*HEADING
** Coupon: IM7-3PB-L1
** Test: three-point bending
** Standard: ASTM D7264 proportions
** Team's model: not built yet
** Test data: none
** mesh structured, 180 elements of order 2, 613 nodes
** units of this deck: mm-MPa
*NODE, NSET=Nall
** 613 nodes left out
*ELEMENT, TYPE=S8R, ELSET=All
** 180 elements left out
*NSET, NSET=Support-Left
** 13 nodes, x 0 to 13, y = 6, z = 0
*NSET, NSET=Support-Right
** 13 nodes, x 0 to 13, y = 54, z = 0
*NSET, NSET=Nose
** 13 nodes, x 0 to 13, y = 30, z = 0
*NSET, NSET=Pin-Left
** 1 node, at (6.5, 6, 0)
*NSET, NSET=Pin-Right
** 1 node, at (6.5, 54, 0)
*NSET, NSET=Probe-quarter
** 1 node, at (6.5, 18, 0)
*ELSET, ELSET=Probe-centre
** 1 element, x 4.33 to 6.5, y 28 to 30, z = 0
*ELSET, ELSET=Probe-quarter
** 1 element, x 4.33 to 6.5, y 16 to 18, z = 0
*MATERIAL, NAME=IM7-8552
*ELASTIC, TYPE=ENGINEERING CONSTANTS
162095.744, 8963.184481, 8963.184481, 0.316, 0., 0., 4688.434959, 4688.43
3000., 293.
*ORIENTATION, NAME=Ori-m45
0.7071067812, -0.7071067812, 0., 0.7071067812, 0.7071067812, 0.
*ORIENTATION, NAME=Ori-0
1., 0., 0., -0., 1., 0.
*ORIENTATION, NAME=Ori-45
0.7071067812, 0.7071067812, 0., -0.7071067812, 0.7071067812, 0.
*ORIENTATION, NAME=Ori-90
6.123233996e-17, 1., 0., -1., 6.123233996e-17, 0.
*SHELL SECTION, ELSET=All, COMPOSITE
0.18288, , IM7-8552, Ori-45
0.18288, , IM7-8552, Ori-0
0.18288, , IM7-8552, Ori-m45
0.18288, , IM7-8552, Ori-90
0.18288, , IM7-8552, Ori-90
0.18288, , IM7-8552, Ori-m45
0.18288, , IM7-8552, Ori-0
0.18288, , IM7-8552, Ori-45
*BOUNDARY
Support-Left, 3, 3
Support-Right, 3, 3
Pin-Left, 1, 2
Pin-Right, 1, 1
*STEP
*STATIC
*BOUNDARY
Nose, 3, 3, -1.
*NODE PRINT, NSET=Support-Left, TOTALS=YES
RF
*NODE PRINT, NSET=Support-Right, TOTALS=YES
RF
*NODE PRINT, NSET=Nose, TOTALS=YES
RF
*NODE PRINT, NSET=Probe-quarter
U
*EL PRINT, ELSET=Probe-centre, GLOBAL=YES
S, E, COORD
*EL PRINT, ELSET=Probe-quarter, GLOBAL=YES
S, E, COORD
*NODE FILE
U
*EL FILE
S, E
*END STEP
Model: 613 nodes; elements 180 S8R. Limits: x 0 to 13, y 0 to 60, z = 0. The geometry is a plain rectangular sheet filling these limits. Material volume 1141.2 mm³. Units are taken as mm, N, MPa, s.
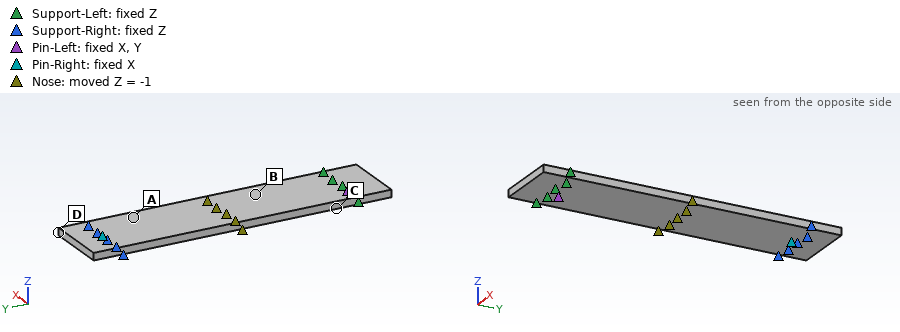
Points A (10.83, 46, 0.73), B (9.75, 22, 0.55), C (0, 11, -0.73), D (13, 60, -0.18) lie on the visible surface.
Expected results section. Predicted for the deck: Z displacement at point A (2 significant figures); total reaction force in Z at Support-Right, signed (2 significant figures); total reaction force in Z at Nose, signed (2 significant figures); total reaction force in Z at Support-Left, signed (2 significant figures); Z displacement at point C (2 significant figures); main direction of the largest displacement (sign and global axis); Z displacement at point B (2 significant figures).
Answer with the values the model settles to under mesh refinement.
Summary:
-0.49 mm
21 N
-43 N
21 N
-0.32 mm
-Z
-0.84 mm
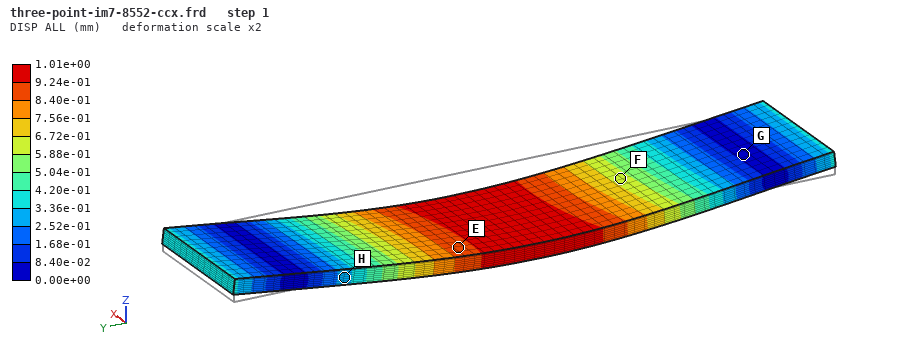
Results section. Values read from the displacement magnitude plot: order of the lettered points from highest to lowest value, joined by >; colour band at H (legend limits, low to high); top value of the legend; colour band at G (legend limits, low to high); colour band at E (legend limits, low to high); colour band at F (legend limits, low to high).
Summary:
E > F > H > G
2.52e-01 to 3.36e-01 mm
1.01e+00 mm
0.00e+00 to 8.40e-02 mm
8.40e-01 to 9.24e-01 mm
5.88e-01 to 6.72e-01 mm
